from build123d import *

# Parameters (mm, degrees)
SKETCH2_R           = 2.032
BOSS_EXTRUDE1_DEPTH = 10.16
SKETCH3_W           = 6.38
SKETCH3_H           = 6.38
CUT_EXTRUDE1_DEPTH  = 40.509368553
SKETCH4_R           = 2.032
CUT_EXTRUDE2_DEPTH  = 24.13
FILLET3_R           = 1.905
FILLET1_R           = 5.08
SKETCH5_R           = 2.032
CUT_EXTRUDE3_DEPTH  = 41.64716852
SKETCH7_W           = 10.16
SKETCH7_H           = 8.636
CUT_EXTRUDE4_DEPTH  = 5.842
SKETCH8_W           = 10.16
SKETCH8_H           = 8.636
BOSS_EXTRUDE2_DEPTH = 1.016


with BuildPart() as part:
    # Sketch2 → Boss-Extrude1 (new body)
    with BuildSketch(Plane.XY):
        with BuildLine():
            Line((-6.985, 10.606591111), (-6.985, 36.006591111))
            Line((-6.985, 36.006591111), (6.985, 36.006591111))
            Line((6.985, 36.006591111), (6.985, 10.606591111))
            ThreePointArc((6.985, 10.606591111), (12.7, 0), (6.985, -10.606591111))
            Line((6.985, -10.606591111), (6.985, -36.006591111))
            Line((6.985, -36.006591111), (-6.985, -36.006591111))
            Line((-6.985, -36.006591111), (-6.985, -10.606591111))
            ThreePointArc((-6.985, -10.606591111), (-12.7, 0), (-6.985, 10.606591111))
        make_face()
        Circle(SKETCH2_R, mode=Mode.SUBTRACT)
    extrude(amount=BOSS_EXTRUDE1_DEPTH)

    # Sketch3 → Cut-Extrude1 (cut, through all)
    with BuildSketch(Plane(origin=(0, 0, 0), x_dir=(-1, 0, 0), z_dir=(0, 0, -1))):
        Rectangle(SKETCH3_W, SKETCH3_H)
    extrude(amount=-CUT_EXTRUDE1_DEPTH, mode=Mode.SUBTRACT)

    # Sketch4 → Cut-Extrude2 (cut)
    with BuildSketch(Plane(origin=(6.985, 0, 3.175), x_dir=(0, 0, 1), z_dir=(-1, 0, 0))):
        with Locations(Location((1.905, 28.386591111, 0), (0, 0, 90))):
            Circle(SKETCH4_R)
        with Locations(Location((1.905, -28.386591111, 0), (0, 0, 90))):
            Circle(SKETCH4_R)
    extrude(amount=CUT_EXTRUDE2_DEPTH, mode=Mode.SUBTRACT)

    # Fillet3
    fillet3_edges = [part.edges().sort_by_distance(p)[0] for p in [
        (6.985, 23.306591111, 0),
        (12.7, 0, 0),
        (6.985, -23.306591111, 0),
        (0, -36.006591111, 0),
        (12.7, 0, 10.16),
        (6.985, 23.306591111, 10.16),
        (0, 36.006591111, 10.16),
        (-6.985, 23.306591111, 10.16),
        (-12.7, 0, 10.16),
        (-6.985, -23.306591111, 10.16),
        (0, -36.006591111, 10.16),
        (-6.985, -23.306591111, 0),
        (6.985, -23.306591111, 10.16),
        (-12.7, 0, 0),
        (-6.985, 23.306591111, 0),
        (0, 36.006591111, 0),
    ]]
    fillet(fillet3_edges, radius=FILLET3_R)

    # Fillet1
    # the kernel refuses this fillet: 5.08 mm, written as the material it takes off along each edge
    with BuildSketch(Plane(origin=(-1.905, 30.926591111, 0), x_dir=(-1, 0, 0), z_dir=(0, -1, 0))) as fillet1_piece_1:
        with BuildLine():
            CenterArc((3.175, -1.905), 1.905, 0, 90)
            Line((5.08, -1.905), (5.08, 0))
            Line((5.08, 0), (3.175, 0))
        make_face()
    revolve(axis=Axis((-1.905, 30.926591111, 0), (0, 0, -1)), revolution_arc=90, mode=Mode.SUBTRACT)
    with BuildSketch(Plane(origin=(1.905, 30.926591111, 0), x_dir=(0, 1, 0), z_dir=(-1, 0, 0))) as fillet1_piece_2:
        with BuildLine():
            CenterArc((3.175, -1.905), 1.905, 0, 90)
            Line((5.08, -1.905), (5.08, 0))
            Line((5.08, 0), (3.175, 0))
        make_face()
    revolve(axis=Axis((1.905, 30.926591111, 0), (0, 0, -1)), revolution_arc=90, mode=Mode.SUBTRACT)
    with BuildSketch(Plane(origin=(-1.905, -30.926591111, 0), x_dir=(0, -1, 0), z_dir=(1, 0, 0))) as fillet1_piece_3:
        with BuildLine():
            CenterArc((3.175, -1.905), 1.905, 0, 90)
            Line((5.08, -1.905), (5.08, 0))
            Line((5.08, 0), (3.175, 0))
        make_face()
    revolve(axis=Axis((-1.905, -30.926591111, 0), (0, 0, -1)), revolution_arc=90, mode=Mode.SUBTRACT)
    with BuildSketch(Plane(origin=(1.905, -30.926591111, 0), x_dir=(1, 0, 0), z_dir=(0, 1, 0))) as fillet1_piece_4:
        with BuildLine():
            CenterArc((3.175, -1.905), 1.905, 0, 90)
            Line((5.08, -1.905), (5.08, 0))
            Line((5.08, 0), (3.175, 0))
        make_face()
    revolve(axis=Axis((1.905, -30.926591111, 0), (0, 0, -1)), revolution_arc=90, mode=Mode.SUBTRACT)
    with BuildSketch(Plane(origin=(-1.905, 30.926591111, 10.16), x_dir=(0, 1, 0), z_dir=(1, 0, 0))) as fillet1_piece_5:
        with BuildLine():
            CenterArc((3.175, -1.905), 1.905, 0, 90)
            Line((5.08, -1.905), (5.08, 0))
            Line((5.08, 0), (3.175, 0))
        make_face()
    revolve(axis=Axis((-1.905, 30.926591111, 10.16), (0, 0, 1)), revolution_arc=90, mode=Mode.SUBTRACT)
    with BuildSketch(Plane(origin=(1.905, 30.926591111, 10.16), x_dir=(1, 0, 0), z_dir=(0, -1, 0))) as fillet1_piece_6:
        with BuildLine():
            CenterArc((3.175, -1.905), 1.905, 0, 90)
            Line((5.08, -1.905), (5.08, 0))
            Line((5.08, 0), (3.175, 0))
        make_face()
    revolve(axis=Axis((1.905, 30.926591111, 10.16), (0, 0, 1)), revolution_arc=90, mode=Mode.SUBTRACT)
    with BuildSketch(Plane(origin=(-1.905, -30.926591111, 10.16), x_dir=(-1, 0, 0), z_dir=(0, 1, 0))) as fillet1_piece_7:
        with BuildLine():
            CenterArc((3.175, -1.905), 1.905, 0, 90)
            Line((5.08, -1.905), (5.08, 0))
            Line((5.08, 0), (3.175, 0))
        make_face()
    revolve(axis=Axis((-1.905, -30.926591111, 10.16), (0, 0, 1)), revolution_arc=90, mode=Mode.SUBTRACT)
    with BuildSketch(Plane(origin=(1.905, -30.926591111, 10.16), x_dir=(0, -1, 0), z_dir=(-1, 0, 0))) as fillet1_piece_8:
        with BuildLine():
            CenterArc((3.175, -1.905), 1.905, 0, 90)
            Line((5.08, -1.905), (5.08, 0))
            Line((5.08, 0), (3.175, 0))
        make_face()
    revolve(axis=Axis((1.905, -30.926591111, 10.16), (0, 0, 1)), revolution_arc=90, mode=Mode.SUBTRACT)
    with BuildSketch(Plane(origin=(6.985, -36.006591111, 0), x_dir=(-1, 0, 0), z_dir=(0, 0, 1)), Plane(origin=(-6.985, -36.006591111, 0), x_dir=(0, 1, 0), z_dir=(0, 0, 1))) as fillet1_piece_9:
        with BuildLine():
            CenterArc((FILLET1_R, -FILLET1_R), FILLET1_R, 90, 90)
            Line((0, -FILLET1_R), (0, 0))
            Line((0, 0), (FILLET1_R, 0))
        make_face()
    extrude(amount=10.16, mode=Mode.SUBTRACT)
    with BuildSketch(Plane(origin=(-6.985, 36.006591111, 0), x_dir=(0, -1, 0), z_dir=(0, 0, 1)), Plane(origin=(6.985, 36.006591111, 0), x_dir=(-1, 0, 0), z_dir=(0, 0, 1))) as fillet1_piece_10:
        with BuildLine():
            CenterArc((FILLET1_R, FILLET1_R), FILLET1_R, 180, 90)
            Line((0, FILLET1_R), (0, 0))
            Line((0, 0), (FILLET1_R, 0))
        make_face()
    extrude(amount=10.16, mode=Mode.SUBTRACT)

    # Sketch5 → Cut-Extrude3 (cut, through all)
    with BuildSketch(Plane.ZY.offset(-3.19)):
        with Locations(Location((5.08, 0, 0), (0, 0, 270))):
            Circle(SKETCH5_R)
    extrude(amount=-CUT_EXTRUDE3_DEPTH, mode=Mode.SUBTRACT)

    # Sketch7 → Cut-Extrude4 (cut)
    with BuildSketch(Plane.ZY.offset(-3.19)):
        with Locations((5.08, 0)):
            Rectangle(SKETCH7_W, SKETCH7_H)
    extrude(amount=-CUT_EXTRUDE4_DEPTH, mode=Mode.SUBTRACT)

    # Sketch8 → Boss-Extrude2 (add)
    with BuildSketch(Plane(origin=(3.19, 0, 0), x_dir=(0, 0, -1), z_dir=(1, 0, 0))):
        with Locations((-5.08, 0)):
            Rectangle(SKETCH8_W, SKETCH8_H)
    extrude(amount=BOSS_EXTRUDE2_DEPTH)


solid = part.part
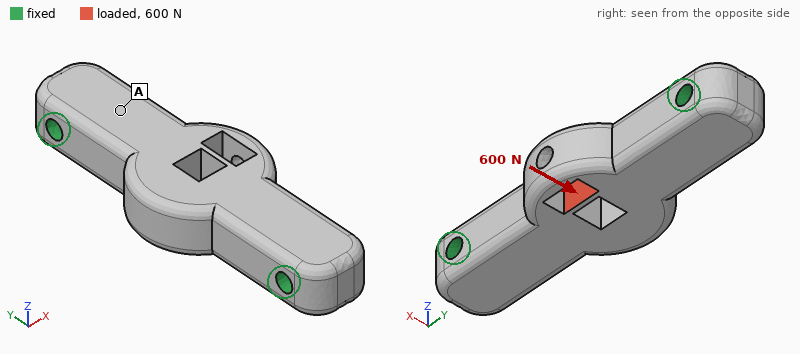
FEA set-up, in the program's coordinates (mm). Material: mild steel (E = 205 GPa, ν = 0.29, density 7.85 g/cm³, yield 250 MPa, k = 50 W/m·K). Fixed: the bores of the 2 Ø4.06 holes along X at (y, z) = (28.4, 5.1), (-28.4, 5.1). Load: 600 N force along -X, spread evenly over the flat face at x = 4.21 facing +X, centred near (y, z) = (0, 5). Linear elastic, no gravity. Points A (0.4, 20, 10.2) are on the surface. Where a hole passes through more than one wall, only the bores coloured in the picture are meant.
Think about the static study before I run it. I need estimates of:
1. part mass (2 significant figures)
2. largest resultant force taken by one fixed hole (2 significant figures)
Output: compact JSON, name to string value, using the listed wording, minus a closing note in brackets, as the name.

{"part mass": "80 g", "largest resultant force taken by one fixed hole": "300 N"}
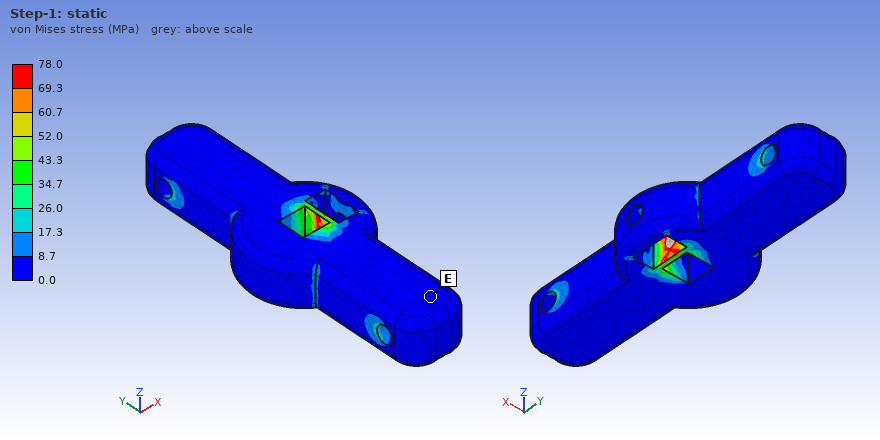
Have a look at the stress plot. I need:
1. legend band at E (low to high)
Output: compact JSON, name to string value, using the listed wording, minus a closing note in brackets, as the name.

{"legend band at E": "0.0 to 8.7 MPa"}
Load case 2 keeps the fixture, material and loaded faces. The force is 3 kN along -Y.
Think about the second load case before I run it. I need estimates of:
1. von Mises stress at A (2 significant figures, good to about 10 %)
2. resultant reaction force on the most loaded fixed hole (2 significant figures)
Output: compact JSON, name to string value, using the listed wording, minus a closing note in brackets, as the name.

{"von Mises stress at A": "12 MPa", "resultant reaction force on the most loaded fixed hole": "1.5 kN"}
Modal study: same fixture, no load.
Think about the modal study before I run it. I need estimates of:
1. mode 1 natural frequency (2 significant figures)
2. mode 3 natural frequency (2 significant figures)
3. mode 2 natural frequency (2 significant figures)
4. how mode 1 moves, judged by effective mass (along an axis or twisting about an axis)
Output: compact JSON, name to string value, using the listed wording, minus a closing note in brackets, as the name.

{"mode 1 natural frequency": "11 kHz", "mode 3 natural frequency": "18 kHz", "mode 2 natural frequency": "18 kHz", "how mode 1 moves, judged by effective mass": "along Z"}
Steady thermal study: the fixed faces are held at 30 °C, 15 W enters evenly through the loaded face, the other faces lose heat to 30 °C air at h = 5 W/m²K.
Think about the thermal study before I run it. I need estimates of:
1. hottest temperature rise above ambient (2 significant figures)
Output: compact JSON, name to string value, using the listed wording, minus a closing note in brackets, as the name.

{"hottest temperature rise above ambient": "57 K"}
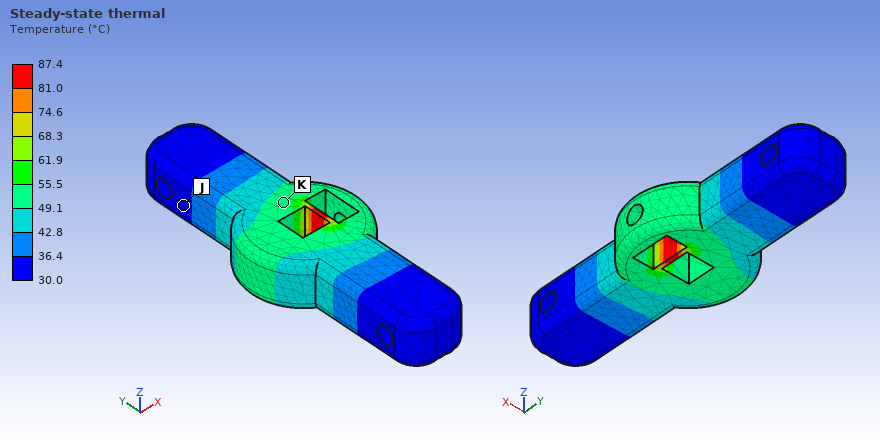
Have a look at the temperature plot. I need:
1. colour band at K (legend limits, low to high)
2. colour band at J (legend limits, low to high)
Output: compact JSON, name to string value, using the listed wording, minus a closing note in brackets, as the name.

{"colour band at K": "49.1 to 55.5 °C", "colour band at J": "30.0 to 36.4 °C"}
